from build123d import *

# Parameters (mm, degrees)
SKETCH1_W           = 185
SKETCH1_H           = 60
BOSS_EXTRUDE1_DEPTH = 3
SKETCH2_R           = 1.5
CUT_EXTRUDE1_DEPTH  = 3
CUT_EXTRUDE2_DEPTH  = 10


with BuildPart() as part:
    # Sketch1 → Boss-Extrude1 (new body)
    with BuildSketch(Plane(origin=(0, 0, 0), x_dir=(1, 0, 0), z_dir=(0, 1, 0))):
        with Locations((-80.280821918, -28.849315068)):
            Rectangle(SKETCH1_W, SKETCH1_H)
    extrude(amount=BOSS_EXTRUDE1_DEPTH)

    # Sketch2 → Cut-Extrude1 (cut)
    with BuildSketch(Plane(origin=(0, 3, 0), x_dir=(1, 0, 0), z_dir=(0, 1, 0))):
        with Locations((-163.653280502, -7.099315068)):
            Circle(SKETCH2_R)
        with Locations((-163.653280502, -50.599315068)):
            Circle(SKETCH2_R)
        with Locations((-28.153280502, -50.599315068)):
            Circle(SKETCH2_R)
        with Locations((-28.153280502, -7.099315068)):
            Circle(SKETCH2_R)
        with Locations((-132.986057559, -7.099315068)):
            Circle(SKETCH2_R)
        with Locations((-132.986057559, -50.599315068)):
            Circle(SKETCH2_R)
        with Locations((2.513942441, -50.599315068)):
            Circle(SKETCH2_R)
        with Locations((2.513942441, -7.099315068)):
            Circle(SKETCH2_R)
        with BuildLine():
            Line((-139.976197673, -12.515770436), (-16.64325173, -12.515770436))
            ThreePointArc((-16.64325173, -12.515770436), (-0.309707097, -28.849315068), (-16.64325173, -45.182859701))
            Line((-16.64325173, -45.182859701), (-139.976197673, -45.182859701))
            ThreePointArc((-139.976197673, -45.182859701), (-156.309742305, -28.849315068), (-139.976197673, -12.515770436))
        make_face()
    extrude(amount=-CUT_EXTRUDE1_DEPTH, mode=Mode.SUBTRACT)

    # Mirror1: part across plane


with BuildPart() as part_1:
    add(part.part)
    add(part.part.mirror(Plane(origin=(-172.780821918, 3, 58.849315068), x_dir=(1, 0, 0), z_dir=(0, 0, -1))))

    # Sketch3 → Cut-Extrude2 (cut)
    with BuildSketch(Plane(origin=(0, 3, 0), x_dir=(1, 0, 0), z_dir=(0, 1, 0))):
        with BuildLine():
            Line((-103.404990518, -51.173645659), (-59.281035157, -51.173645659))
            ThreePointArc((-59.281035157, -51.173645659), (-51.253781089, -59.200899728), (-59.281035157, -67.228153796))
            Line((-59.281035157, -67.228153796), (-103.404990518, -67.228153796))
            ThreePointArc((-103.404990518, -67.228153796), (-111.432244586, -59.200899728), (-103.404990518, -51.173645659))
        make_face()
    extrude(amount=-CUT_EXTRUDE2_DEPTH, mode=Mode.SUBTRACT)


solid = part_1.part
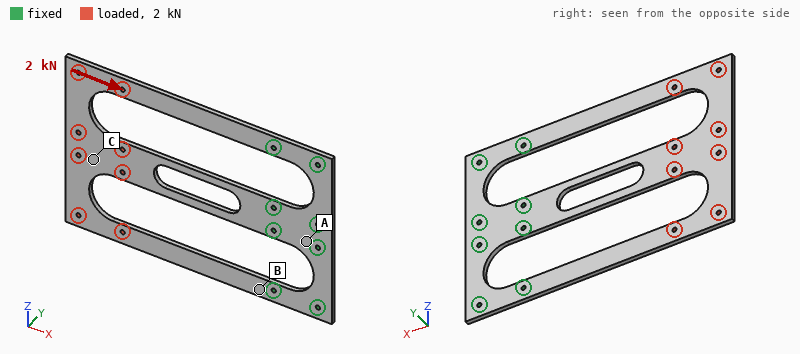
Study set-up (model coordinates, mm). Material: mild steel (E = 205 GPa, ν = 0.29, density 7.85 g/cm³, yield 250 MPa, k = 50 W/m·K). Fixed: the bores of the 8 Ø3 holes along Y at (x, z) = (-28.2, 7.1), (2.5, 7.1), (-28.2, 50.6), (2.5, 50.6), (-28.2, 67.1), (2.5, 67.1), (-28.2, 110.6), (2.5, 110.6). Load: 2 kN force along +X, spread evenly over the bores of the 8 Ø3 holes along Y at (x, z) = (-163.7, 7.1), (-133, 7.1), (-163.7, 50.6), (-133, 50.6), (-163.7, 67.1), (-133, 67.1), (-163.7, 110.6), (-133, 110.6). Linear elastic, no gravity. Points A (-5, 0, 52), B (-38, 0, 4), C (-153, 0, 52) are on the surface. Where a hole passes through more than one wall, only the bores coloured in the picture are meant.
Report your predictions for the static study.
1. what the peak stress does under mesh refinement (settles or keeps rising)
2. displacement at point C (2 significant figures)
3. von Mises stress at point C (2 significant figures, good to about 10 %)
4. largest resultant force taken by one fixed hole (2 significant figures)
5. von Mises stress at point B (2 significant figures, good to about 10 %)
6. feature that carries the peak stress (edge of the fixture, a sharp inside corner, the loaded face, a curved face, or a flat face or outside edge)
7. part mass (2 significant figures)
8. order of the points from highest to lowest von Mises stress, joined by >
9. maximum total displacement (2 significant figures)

keeps rising
12 µm
7.5 MPa
480 N
14 MPa
edge of the fixture
270 g
B > C > A
12 µm
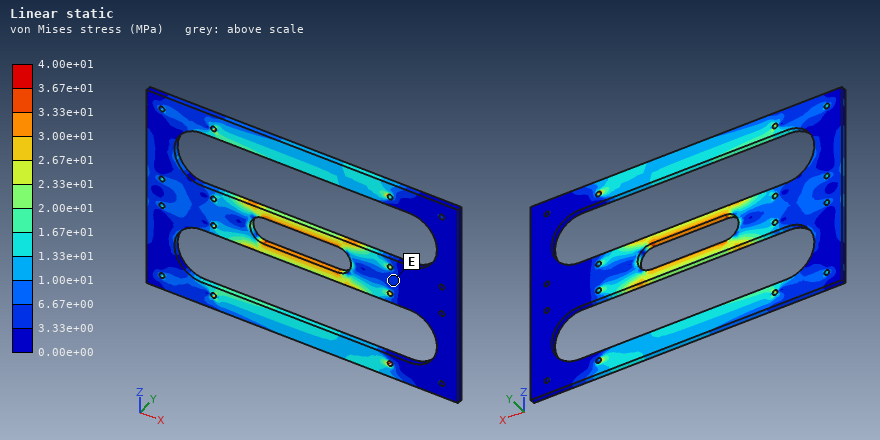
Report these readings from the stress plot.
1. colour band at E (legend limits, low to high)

3.33e+00 to 6.67e+00 MPa
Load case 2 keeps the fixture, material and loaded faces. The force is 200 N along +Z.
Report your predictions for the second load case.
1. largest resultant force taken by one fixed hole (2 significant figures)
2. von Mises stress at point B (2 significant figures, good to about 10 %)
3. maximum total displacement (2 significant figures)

270 N
10 MPa
91 µm
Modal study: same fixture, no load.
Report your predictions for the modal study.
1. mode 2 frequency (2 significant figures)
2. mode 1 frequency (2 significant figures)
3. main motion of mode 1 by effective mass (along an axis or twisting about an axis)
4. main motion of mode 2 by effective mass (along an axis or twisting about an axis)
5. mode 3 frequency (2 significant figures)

250 Hz
87 Hz
along Y
twisting about X
650 Hz
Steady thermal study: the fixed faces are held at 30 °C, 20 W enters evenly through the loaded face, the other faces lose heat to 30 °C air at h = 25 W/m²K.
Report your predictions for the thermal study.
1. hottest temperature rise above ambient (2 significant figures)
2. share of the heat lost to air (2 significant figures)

67 K
91 %
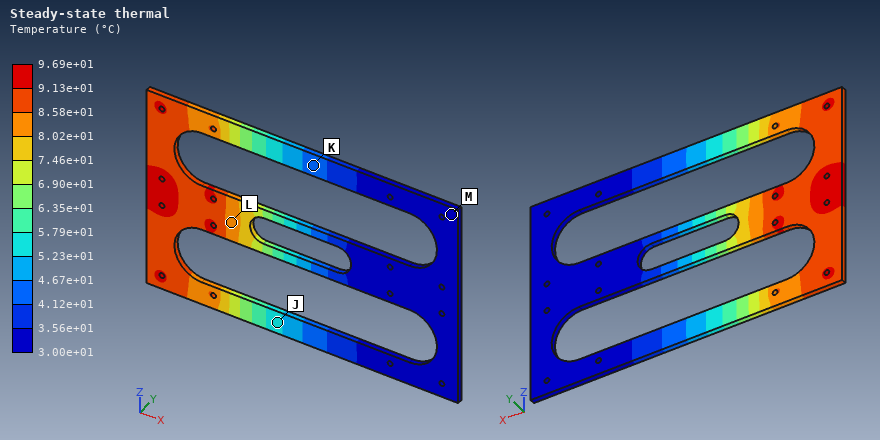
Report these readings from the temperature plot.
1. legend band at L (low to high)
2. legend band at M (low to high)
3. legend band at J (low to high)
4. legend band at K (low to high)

8.02e+01 to 8.58e+01 °C
3.00e+01 to 3.56e+01 °C
5.23e+01 to 5.79e+01 °C
4.12e+01 to 4.67e+01 °C
